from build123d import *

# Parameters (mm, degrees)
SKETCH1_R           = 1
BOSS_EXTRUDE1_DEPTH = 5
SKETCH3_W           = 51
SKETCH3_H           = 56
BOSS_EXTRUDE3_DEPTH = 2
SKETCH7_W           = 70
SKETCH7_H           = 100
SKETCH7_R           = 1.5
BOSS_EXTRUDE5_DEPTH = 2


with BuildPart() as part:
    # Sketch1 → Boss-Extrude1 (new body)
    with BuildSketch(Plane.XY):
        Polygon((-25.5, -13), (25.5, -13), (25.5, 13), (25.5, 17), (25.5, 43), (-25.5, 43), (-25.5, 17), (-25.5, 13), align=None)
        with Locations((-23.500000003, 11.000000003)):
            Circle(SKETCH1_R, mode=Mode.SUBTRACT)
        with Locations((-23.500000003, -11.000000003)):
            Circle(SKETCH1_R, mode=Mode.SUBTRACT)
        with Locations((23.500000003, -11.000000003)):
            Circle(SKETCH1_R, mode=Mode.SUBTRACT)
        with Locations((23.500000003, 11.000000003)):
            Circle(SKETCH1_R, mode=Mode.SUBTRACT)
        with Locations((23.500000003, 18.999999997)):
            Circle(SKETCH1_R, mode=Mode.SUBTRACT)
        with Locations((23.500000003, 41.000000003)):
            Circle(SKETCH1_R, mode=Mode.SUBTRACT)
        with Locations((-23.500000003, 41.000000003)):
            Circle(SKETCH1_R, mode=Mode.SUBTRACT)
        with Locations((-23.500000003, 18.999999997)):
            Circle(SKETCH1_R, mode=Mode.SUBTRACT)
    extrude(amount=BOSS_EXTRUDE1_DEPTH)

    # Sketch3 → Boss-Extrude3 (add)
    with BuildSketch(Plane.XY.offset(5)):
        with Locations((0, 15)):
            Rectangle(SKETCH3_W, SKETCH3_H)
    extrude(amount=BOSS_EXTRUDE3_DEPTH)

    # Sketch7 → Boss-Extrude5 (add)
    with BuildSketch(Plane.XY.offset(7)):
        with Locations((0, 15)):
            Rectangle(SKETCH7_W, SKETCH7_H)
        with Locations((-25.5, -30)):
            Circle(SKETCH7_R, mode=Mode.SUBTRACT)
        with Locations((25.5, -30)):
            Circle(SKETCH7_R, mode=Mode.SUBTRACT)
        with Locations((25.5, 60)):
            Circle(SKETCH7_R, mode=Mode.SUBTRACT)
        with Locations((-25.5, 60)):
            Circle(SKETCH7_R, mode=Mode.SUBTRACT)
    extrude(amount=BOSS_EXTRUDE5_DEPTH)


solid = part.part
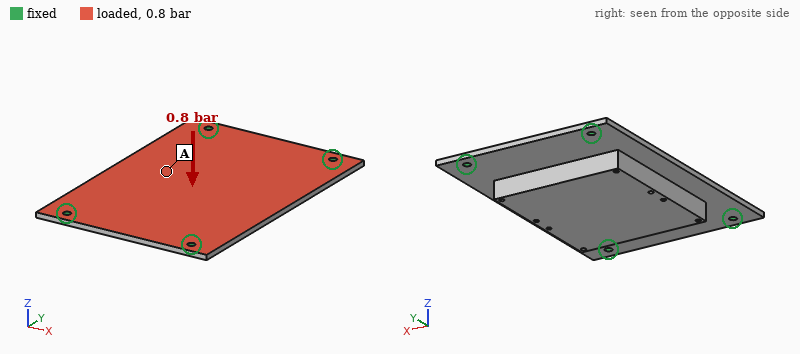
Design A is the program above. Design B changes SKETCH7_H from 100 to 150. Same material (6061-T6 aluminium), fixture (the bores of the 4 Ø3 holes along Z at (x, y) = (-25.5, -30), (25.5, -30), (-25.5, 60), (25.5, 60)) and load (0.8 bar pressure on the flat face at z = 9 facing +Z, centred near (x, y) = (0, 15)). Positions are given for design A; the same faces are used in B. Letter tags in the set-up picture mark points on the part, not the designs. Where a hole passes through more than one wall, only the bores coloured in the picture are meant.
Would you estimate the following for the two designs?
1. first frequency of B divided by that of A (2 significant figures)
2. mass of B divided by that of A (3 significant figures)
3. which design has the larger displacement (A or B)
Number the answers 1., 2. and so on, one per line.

1. 0.96
2. 1.21
3. B
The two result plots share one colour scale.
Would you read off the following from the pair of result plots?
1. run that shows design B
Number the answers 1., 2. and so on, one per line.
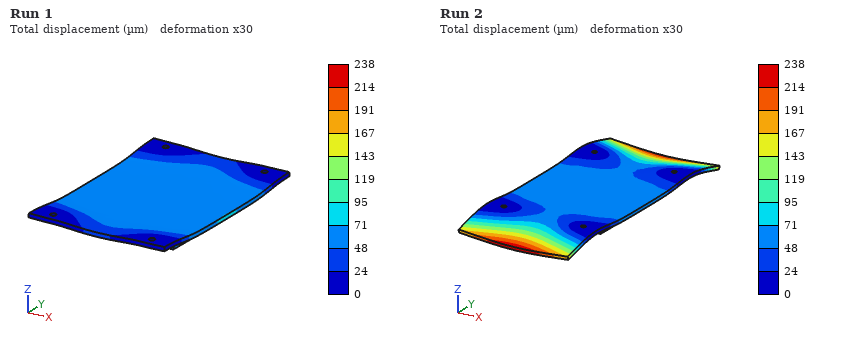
1. Run 2
